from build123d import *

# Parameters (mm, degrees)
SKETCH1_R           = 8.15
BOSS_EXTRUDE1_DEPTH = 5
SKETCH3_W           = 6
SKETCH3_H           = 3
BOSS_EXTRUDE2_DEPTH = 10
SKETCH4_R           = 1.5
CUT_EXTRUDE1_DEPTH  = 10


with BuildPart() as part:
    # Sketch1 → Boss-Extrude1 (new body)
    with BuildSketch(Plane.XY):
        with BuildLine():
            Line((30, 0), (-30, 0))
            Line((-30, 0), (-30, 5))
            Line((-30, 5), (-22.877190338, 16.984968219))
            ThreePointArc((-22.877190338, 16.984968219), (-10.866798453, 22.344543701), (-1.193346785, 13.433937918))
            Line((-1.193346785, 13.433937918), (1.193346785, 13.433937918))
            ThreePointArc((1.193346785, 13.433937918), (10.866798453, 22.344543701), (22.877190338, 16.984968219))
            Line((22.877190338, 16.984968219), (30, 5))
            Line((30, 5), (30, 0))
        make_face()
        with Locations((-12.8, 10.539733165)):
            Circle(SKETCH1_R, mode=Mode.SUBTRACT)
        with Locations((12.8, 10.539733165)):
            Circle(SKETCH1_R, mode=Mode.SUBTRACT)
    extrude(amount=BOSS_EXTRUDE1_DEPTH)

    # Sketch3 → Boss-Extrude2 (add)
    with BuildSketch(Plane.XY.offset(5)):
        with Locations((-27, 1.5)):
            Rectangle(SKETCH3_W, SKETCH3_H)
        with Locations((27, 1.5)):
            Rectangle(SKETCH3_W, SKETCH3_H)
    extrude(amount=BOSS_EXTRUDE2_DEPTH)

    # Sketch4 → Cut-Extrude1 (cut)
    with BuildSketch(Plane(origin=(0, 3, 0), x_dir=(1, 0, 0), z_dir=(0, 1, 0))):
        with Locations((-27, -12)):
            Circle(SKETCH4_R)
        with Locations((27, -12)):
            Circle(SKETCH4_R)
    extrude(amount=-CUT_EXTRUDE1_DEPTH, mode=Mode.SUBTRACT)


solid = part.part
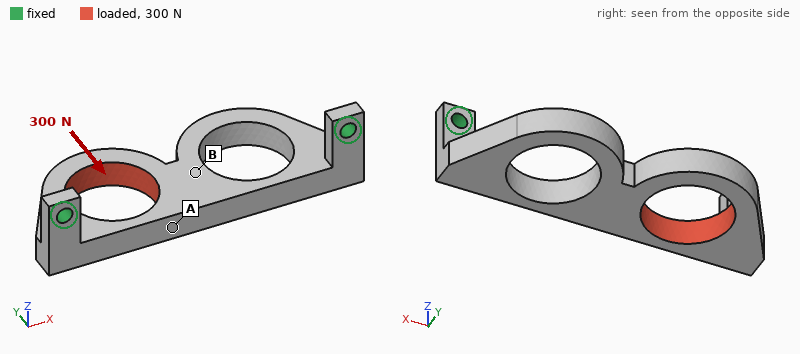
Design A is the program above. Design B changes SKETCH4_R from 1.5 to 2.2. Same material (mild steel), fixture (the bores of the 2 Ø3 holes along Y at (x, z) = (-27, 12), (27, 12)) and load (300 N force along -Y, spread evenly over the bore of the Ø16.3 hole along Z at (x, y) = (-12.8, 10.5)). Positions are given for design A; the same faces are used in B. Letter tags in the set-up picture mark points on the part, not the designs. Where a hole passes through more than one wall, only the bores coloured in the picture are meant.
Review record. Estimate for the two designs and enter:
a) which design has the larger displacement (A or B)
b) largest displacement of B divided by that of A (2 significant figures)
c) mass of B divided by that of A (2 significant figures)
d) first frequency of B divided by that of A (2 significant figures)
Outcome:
A
0.82
0.99
1.1
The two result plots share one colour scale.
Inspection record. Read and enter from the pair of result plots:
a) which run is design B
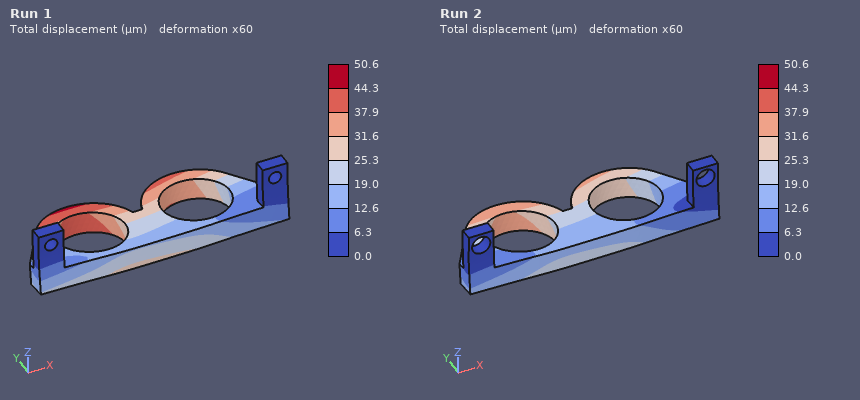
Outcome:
Run 2
